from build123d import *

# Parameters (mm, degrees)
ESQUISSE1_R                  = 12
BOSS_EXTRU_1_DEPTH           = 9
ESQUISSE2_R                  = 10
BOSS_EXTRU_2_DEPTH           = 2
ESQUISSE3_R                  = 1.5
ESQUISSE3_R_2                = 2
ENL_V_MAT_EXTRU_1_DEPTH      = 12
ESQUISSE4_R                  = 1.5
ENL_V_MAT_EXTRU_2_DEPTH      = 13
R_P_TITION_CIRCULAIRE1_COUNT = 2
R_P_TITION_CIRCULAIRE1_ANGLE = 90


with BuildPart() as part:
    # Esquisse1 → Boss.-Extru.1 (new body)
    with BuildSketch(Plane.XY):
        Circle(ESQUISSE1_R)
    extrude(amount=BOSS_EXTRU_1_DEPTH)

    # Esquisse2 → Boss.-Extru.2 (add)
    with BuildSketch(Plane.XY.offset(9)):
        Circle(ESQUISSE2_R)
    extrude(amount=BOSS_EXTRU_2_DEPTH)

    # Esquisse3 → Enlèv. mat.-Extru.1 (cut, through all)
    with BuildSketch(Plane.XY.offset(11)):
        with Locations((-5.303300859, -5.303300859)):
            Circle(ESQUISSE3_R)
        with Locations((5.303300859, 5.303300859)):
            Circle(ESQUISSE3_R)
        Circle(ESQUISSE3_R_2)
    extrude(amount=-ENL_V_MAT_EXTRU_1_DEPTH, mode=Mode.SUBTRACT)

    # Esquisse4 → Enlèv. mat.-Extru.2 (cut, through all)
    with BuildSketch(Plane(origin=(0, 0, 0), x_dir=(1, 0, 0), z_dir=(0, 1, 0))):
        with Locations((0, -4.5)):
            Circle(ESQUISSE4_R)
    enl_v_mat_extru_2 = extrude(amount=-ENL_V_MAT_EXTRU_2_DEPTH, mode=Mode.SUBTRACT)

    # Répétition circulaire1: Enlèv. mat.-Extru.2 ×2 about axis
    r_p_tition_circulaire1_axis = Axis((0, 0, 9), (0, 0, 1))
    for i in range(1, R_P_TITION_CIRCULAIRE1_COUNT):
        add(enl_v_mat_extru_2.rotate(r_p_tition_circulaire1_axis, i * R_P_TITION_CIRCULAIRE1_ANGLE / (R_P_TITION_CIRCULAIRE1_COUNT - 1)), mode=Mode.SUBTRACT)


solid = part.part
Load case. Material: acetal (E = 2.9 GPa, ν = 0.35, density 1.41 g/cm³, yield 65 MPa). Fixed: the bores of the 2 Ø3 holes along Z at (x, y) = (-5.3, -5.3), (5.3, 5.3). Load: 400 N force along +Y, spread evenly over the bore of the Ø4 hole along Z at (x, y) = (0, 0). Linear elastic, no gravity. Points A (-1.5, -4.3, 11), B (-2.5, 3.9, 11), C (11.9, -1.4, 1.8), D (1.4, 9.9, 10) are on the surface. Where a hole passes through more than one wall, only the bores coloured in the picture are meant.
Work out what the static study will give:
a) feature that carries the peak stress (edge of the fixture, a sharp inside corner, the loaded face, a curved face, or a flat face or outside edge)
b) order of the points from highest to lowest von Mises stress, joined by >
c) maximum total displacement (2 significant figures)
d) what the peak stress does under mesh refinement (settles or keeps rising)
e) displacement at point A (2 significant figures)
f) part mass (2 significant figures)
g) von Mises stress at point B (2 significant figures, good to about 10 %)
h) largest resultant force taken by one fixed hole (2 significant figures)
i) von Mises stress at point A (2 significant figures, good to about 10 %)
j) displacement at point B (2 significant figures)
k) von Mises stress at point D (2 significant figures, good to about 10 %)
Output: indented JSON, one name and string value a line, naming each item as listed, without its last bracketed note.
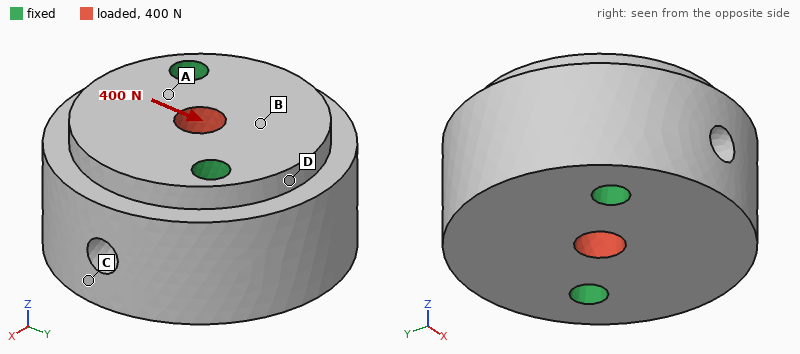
{
  "feature that carries the peak stress": "a sharp inside corner",
  "order of the points from highest to lowest von Mises stress, joined by >": "A > B > D > C",
  "maximum total displacement": "8.8 µm",
  "what the peak stress does under mesh refinement": "keeps rising",
  "displacement at point A": "5.0 µm",
  "part mass": "6.0 g",
  "von Mises stress at point B": "1.8 MPa",
  "largest resultant force taken by one fixed hole": "210 N",
  "von Mises stress at point A": "2.5 MPa",
  "displacement at point B": "6.3 µm",
  "von Mises stress at point D": "0.93 MPa"
}
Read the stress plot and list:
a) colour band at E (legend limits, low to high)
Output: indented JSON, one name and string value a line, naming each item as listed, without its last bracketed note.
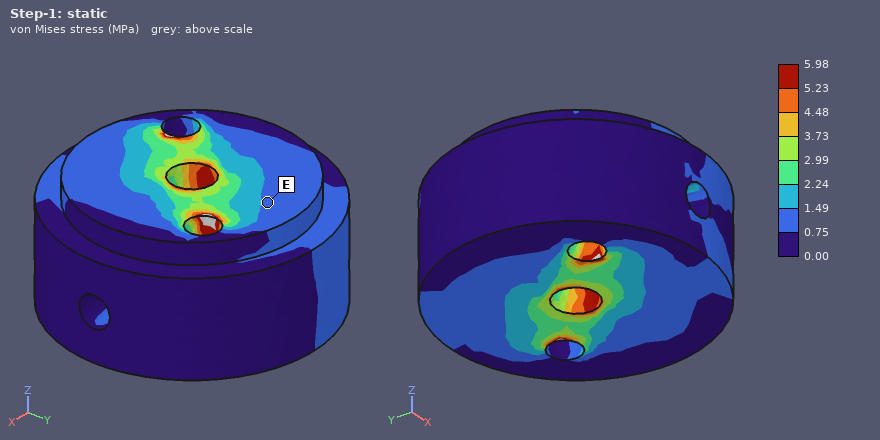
{
  "colour band at E": "0.75 to 1.49 MPa"
}
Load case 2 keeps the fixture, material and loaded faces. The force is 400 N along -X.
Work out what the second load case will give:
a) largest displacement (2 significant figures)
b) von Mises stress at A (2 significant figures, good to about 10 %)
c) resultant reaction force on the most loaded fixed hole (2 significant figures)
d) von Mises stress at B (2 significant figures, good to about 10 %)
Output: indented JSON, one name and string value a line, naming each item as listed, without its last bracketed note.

{
  "largest displacement": "8.8 µm",
  "von Mises stress at A": "2.1 MPa",
  "resultant reaction force on the most loaded fixed hole": "210 N",
  "von Mises stress at B": "1.7 MPa"
}
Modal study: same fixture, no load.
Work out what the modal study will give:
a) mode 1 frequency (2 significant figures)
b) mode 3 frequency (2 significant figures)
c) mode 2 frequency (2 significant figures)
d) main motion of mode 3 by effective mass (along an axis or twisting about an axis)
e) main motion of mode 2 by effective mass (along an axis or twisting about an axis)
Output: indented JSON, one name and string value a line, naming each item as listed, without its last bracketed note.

{
  "mode 1 frequency": "12 kHz",
  "mode 3 frequency": "18 kHz",
  "mode 2 frequency": "14 kHz",
  "main motion of mode 3 by effective mass": "twisting about Z",
  "main motion of mode 2 by effective mass": "along Z"
}
